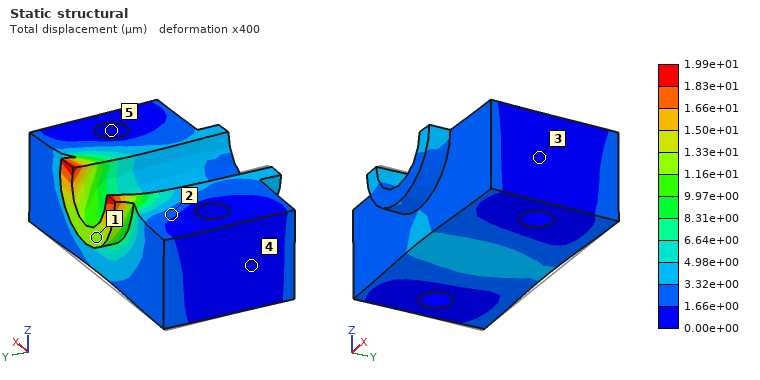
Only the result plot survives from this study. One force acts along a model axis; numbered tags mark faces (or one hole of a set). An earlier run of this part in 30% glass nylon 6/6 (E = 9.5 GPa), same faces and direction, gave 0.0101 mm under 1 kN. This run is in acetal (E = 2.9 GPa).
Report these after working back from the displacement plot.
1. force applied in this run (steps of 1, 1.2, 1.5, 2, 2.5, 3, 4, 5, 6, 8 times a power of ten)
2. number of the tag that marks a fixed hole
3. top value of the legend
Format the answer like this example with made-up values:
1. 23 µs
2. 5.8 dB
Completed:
1. 600 N
2. 5
3. 1.99e+01 µm
